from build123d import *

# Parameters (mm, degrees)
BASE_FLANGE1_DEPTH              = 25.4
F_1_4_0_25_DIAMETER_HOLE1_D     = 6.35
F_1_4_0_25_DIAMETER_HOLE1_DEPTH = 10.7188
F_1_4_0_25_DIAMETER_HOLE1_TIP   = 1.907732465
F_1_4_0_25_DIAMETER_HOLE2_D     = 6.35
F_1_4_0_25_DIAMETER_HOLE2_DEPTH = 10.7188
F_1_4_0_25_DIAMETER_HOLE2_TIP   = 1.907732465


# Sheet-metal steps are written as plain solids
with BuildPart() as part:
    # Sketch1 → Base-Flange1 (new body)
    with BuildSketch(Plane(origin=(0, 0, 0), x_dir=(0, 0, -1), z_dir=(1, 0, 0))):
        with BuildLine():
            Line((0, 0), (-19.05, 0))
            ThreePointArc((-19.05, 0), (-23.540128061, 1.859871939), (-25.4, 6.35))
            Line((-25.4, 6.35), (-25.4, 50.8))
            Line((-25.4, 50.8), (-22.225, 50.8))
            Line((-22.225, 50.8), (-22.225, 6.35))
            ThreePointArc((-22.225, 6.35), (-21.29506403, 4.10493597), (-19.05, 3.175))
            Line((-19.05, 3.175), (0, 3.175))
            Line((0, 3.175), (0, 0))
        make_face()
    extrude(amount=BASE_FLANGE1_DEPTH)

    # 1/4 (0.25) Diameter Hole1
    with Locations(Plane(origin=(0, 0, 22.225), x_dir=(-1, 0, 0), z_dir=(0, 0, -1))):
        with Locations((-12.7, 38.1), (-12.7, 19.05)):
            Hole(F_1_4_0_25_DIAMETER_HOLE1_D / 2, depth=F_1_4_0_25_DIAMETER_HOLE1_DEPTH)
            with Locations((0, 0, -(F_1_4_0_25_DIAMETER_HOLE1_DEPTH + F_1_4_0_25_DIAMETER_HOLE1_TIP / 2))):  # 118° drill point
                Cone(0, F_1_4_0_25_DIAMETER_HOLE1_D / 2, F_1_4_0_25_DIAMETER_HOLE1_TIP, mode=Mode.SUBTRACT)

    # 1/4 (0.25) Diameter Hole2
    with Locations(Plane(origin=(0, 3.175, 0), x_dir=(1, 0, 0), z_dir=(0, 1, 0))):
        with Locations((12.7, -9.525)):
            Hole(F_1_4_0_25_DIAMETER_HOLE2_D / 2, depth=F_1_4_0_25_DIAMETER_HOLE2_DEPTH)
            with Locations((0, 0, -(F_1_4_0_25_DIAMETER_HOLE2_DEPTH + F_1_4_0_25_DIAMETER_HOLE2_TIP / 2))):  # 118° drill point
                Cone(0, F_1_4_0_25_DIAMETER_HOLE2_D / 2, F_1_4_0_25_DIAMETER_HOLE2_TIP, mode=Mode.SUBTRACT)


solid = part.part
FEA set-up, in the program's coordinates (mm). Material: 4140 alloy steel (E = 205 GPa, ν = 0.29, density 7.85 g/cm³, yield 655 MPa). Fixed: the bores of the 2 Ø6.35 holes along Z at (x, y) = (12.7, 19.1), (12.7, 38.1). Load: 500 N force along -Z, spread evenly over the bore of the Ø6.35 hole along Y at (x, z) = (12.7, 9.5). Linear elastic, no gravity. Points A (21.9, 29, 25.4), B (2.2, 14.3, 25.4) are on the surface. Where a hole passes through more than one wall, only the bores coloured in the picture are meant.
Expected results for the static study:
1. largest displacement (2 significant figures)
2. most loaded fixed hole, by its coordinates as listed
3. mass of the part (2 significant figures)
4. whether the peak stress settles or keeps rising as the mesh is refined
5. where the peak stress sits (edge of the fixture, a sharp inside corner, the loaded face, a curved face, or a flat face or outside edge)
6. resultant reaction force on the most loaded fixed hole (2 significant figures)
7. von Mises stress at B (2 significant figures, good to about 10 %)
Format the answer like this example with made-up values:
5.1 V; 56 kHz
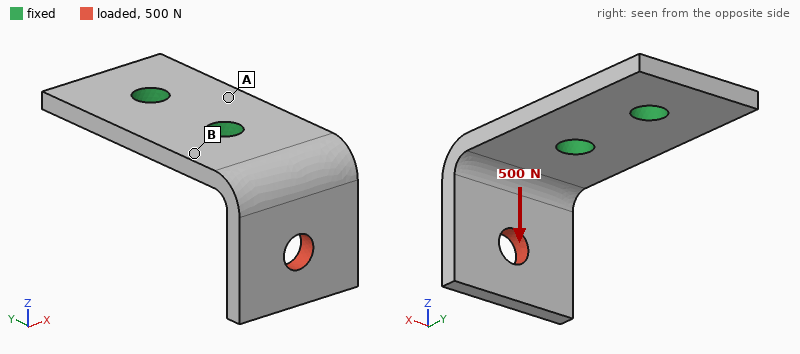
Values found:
0.13 mm; (12.7, 19.1); 43 g; keeps rising; edge of the fixture; 570 N; 99 MPa
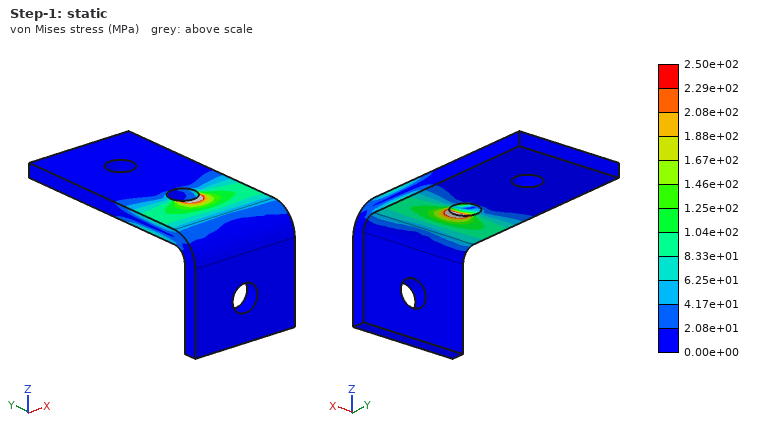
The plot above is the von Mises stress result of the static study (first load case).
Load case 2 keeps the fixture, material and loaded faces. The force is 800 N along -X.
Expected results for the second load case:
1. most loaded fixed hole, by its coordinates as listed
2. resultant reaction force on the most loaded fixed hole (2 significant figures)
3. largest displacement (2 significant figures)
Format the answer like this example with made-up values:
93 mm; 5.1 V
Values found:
(12.7, 19.1); 1.2 kN; 0.19 mm
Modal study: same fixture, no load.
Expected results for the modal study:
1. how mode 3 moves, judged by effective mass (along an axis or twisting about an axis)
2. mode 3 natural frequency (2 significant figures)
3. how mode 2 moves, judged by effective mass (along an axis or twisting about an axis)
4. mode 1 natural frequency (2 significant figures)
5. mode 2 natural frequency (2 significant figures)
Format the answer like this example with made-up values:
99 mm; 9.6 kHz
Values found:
along Z; 6800 Hz; along X; 2300 Hz; 3400 Hz
